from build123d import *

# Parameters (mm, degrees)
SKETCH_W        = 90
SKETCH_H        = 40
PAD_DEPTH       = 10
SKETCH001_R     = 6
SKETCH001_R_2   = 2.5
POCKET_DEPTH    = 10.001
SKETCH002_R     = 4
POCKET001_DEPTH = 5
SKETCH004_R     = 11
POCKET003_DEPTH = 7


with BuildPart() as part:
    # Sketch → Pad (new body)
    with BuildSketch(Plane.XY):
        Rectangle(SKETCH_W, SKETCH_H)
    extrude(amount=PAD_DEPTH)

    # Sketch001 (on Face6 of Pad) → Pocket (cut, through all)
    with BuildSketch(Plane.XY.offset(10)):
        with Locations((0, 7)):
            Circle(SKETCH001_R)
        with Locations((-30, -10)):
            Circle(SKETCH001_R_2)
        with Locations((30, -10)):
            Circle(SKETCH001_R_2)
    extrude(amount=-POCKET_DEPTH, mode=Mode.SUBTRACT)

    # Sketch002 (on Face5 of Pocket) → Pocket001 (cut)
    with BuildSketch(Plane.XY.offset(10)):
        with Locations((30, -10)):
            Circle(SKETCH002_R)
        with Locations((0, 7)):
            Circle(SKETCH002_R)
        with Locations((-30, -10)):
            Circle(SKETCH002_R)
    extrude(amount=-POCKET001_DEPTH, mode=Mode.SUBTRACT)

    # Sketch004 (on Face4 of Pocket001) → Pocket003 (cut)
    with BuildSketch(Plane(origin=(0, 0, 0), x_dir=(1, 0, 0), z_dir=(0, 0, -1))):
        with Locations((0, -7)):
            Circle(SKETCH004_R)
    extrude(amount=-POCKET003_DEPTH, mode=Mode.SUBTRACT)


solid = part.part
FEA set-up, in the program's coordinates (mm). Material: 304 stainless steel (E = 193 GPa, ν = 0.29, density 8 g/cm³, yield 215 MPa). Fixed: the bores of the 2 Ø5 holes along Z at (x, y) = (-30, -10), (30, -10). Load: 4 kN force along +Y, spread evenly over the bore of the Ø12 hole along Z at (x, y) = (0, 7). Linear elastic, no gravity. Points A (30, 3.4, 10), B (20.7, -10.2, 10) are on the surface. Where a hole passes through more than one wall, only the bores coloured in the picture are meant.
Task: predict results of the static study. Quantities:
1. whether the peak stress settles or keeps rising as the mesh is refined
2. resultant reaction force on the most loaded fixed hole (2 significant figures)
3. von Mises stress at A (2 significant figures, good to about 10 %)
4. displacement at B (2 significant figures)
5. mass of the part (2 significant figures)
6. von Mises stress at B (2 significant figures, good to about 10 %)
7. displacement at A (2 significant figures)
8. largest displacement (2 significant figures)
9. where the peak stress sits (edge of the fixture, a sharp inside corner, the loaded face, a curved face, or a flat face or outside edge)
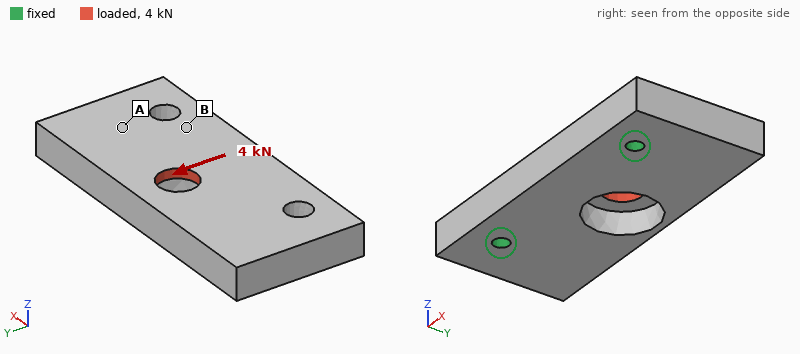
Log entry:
keeps rising
2.1 kN
14 MPa
6.4 µm
260 g
29 MPa
9.4 µm
28 µm
edge of the fixture
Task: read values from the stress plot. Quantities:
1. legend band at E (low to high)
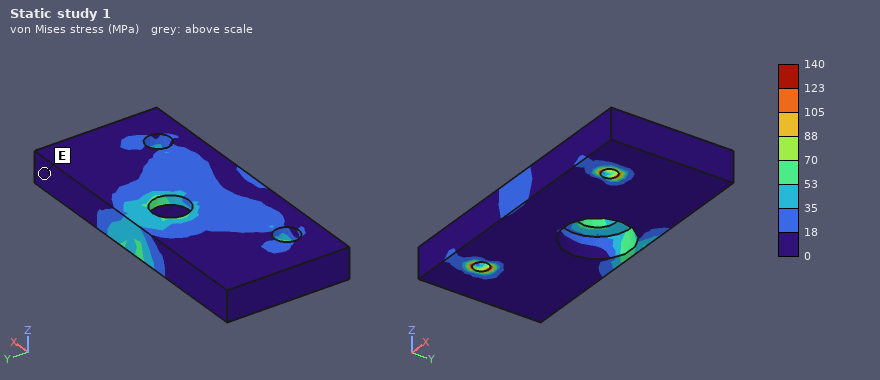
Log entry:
0 to 18 MPa
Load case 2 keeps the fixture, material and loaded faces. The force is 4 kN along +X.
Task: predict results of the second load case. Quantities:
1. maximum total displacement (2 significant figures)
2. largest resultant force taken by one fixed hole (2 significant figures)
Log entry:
5.9 µm
2.3 kN
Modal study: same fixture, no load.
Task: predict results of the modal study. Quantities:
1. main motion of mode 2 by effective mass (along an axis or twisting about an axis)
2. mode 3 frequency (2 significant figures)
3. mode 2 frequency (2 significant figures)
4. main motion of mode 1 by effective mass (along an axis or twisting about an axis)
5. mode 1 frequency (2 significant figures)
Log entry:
twisting about Y
7900 Hz
6300 Hz
along Z
3800 Hz
